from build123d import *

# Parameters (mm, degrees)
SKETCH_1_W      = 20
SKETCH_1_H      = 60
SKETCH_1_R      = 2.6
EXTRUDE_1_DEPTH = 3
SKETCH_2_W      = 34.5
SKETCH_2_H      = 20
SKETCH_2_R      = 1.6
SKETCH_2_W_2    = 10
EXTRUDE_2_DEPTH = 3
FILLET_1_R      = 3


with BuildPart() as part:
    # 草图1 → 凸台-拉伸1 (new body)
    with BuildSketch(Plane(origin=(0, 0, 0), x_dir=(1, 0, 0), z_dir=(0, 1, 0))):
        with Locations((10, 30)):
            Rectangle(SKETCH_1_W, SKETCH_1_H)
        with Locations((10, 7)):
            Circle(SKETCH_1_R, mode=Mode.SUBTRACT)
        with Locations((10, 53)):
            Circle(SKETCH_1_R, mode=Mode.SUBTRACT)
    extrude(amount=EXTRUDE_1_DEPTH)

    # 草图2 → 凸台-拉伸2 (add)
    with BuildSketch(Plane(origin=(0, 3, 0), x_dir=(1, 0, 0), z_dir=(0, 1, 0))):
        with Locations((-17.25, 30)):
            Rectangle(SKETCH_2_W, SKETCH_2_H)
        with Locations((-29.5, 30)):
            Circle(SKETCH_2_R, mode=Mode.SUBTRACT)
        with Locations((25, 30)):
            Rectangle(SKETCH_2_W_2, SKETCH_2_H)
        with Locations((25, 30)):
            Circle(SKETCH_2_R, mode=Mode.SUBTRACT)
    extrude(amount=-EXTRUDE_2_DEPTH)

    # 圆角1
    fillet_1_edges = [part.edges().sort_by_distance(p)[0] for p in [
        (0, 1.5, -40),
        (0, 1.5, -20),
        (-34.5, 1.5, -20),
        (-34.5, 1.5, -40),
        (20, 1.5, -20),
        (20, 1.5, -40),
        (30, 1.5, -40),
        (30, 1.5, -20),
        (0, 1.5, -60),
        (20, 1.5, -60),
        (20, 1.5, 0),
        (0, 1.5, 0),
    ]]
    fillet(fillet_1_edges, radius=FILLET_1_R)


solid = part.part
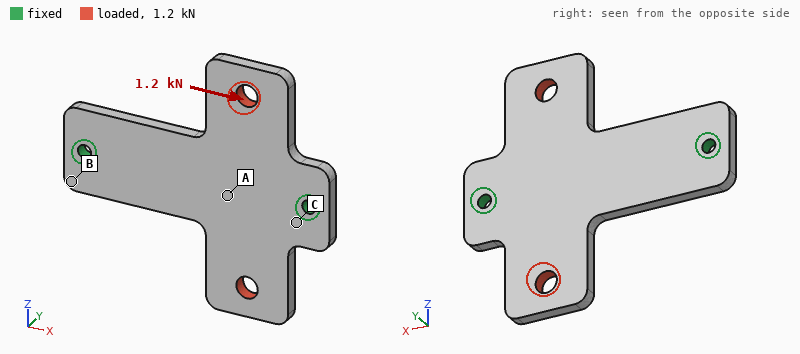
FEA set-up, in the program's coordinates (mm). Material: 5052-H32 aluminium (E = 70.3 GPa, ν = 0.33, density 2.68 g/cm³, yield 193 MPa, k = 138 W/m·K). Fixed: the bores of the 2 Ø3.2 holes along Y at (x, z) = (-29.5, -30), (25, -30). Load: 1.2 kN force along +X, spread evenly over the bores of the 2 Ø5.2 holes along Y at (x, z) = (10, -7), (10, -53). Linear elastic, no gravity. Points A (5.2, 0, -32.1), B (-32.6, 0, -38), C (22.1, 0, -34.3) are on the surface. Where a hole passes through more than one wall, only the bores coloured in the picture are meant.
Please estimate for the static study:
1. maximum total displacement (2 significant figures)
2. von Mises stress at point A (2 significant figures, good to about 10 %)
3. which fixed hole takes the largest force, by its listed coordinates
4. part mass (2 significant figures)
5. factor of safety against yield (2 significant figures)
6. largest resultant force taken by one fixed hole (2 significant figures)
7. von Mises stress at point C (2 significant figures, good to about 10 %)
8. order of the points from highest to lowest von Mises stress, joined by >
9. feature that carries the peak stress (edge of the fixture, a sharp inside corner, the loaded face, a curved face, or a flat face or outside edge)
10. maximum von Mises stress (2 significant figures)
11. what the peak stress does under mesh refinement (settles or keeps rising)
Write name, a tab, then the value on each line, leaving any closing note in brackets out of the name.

maximum total displacement	21 µm
von Mises stress at point A	12 MPa
which fixed hole takes the largest force, by its listed coordinates	(25, -30)
part mass	16 g
factor of safety against yield	2.8
largest resultant force taken by one fixed hole	800 N
von Mises stress at point C	23 MPa
order of the points from highest to lowest von Mises stress, joined by >	C > A > B
feature that carries the peak stress	a curved face
maximum von Mises stress	68 MPa
what the peak stress does under mesh refinement	settles
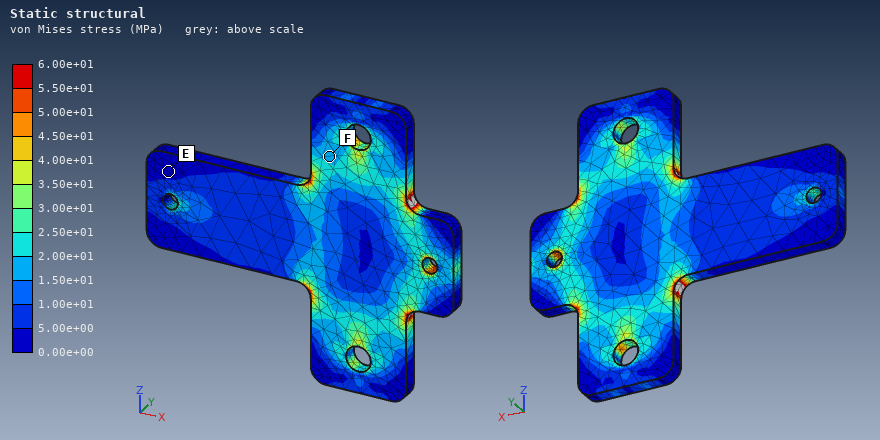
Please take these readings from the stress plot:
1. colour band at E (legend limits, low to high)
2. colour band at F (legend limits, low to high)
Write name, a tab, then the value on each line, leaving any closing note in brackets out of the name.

colour band at E	0.00e+00 to 5.00e+00 MPa
colour band at F	1.50e+01 to 2.00e+01 MPa
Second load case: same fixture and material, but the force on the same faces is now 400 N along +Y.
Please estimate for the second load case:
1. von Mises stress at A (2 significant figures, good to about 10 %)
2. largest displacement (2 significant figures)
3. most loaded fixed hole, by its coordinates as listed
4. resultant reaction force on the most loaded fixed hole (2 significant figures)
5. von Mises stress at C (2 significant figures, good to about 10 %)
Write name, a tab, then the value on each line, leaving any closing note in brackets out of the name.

von Mises stress at A	76 MPa
largest displacement	0.33 mm
most loaded fixed hole, by its coordinates as listed	(25, -30)
resultant reaction force on the most loaded fixed hole	320 N
von Mises stress at C	78 MPa
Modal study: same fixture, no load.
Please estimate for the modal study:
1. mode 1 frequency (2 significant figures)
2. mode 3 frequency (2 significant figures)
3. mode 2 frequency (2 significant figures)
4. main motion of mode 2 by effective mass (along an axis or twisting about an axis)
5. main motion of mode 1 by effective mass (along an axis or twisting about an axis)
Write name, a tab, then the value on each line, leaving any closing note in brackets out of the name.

mode 1 frequency	2200 Hz
mode 3 frequency	5500 Hz
mode 2 frequency	2900 Hz
main motion of mode 2 by effective mass	along Y
main motion of mode 1 by effective mass	twisting about X
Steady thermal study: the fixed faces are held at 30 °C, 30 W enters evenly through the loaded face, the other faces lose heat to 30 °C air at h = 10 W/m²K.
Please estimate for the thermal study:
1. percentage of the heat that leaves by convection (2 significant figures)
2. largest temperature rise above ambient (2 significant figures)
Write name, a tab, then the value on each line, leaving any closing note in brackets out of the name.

percentage of the heat that leaves by convection	4.7 %
largest temperature rise above ambient	63 K
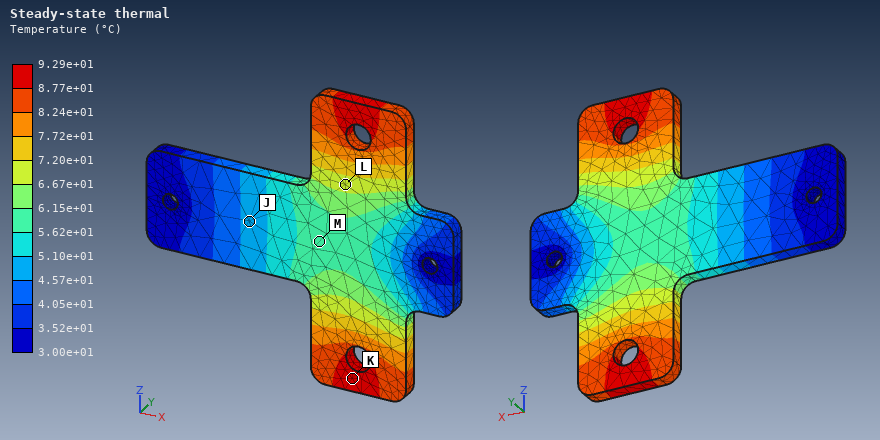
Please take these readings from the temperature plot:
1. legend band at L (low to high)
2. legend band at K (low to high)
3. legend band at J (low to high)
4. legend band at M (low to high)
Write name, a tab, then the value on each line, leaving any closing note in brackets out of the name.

legend band at L	6.67e+01 to 7.20e+01 °C
legend band at K	8.77e+01 to 9.29e+01 °C
legend band at J	4.57e+01 to 5.10e+01 °C
legend band at M	5.62e+01 to 6.15e+01 °C
